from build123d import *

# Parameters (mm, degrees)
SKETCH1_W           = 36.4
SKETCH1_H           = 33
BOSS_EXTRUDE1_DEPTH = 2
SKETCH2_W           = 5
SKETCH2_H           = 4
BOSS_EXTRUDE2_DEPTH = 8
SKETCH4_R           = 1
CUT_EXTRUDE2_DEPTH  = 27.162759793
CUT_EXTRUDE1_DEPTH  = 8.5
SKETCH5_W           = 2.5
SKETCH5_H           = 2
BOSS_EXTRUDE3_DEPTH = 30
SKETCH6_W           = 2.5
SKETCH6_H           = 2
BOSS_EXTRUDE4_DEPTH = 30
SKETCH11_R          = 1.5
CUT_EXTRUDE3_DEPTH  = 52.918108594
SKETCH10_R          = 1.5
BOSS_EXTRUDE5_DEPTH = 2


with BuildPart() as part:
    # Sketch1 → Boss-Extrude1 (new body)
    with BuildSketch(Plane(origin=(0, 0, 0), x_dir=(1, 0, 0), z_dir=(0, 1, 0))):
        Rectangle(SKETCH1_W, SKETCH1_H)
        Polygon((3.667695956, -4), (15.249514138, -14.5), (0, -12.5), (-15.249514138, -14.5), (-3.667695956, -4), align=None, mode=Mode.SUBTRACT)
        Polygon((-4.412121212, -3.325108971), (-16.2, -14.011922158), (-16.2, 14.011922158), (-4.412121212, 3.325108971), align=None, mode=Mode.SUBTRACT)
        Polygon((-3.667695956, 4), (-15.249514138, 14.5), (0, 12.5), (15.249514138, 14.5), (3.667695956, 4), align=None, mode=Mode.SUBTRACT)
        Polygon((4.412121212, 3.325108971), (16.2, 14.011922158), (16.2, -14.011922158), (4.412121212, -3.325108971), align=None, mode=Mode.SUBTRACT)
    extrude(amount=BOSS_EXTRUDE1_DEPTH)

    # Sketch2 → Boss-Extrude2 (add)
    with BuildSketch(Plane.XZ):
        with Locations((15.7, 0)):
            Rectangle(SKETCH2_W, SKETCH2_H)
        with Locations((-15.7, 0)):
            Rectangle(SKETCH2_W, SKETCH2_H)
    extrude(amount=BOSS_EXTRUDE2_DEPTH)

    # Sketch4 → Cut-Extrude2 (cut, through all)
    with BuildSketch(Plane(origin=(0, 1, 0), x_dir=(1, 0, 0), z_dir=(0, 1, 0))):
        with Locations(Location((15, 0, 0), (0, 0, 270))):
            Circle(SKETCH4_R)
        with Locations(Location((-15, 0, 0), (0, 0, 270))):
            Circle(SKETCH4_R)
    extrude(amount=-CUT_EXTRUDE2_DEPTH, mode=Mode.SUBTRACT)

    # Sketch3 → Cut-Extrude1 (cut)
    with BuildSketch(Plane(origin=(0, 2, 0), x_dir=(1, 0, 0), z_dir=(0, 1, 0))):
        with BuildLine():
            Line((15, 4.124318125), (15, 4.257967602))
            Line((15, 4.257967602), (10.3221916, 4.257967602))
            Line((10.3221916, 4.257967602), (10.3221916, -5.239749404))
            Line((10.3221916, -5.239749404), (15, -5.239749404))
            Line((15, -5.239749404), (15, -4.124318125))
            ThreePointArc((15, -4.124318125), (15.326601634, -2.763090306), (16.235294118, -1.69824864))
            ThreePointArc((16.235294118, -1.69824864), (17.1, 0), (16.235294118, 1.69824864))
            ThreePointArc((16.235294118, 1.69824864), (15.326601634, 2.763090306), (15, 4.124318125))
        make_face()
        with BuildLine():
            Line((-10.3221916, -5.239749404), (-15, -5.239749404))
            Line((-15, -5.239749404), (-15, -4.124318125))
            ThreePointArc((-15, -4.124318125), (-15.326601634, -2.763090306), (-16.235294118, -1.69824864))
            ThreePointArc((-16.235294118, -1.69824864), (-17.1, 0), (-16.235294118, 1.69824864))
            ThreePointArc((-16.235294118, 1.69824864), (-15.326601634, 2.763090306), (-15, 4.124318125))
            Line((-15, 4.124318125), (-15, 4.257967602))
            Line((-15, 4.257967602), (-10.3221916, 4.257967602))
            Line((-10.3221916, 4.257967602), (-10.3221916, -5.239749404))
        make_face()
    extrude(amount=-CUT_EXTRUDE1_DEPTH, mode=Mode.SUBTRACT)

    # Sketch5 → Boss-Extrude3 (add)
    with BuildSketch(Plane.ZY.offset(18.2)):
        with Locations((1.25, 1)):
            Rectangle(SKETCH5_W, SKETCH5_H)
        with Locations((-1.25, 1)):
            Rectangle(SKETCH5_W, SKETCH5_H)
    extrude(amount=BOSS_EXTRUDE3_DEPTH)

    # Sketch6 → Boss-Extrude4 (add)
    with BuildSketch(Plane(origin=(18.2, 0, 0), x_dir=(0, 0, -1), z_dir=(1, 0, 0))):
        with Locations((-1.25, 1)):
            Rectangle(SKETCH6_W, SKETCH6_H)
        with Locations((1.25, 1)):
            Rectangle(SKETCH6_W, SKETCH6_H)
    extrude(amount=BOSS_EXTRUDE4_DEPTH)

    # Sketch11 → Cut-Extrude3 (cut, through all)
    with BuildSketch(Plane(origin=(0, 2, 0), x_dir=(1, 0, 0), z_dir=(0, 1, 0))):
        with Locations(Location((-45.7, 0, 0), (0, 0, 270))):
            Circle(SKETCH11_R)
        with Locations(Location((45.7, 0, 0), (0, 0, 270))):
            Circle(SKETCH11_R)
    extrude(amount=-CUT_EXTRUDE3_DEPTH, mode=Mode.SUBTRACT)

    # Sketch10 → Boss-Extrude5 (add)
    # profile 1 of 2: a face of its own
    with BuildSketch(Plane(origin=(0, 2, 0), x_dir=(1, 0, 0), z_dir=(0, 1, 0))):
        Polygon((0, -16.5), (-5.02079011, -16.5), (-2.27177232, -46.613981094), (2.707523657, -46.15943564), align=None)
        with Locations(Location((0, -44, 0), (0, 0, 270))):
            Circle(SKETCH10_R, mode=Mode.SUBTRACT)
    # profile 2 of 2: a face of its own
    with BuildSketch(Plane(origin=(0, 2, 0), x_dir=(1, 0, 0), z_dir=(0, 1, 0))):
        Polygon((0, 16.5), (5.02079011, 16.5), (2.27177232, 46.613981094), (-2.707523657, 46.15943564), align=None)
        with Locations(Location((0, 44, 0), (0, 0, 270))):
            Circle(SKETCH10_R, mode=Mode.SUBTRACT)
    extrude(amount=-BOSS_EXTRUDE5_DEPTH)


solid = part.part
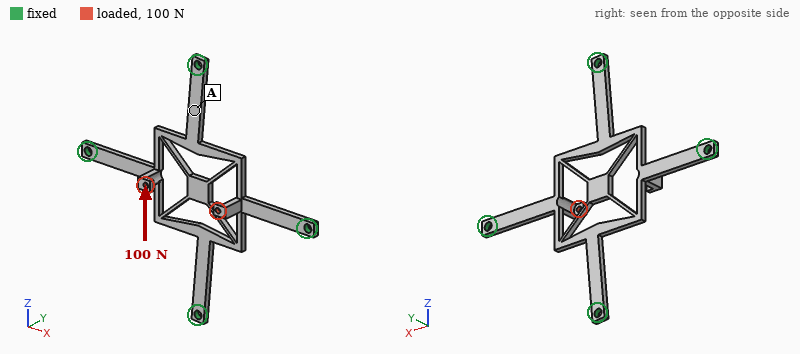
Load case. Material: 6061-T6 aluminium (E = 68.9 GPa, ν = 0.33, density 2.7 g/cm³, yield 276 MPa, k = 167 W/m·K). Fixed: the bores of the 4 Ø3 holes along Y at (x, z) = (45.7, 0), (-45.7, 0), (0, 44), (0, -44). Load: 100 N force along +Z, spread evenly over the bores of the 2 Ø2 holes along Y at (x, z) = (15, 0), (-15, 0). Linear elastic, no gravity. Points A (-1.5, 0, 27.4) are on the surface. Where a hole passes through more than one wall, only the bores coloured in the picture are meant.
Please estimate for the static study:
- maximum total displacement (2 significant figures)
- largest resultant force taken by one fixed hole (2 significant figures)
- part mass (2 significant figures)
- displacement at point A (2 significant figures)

0.28 mm
45 N
5.9 g
0.054 mm
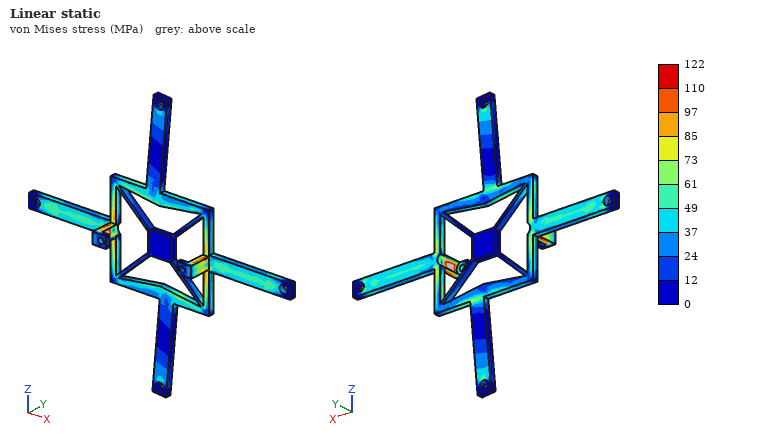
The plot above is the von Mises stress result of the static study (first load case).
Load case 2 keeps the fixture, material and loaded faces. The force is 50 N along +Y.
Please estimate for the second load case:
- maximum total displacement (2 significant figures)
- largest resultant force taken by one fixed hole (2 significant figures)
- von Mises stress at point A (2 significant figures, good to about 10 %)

0.42 mm
14 N
23 MPa
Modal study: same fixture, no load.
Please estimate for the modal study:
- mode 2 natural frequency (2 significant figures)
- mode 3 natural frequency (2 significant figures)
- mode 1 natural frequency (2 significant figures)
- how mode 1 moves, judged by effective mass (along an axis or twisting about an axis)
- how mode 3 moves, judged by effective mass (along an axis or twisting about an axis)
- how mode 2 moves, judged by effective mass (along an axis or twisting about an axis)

2000 Hz
2300 Hz
1200 Hz
along Y
twisting about X
twisting about Z
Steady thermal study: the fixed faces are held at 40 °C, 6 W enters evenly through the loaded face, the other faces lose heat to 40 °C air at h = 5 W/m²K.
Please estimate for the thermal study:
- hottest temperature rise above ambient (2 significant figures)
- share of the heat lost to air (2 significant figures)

64 K
5.5 %
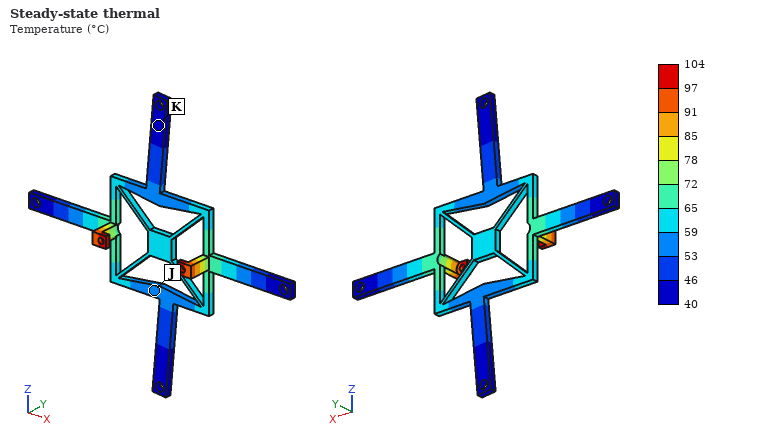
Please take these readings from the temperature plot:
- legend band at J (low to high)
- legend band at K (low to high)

53 to 59 °C
40 to 46 °C
